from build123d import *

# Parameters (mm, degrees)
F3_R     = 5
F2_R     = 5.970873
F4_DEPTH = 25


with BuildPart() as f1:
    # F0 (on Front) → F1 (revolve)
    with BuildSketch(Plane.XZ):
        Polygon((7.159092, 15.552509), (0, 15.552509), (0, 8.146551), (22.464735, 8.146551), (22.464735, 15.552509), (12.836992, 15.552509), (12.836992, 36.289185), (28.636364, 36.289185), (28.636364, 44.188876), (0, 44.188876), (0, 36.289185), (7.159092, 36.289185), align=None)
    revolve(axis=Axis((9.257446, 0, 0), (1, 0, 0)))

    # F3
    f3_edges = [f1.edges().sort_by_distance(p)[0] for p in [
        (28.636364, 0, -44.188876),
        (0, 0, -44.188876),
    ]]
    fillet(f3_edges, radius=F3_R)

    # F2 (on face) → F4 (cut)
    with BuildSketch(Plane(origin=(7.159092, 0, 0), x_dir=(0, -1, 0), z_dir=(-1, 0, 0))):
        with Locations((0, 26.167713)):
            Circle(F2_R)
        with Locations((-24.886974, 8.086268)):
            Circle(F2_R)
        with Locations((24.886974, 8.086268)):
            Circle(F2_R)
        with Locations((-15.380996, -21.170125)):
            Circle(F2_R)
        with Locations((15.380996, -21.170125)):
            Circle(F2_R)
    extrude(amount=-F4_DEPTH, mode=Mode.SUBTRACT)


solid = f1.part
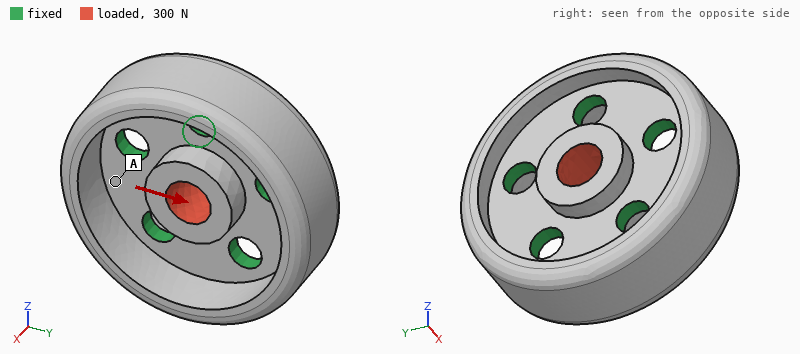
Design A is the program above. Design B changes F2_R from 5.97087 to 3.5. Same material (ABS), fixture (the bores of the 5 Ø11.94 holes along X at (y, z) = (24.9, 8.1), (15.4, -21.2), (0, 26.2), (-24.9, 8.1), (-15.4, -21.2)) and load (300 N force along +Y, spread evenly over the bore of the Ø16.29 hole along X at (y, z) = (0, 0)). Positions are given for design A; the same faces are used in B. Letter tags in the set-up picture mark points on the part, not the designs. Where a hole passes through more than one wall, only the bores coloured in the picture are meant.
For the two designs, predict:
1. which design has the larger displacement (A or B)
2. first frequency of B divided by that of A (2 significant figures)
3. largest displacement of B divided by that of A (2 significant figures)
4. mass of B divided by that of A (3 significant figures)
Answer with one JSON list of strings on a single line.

["B", "0.84", "1.2", "1.03"]
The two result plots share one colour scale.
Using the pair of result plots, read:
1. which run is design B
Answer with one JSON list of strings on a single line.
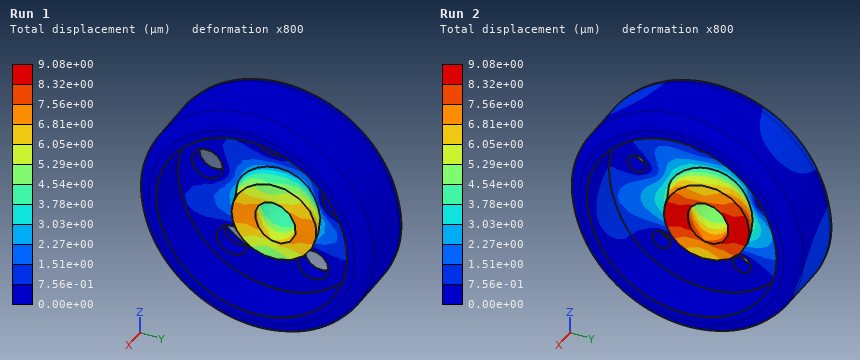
["Run 2"]
